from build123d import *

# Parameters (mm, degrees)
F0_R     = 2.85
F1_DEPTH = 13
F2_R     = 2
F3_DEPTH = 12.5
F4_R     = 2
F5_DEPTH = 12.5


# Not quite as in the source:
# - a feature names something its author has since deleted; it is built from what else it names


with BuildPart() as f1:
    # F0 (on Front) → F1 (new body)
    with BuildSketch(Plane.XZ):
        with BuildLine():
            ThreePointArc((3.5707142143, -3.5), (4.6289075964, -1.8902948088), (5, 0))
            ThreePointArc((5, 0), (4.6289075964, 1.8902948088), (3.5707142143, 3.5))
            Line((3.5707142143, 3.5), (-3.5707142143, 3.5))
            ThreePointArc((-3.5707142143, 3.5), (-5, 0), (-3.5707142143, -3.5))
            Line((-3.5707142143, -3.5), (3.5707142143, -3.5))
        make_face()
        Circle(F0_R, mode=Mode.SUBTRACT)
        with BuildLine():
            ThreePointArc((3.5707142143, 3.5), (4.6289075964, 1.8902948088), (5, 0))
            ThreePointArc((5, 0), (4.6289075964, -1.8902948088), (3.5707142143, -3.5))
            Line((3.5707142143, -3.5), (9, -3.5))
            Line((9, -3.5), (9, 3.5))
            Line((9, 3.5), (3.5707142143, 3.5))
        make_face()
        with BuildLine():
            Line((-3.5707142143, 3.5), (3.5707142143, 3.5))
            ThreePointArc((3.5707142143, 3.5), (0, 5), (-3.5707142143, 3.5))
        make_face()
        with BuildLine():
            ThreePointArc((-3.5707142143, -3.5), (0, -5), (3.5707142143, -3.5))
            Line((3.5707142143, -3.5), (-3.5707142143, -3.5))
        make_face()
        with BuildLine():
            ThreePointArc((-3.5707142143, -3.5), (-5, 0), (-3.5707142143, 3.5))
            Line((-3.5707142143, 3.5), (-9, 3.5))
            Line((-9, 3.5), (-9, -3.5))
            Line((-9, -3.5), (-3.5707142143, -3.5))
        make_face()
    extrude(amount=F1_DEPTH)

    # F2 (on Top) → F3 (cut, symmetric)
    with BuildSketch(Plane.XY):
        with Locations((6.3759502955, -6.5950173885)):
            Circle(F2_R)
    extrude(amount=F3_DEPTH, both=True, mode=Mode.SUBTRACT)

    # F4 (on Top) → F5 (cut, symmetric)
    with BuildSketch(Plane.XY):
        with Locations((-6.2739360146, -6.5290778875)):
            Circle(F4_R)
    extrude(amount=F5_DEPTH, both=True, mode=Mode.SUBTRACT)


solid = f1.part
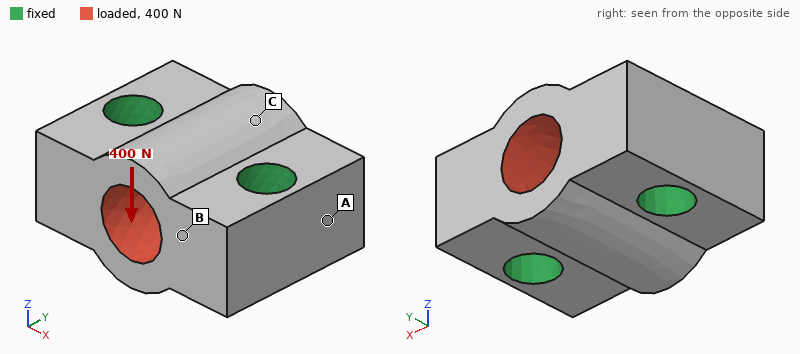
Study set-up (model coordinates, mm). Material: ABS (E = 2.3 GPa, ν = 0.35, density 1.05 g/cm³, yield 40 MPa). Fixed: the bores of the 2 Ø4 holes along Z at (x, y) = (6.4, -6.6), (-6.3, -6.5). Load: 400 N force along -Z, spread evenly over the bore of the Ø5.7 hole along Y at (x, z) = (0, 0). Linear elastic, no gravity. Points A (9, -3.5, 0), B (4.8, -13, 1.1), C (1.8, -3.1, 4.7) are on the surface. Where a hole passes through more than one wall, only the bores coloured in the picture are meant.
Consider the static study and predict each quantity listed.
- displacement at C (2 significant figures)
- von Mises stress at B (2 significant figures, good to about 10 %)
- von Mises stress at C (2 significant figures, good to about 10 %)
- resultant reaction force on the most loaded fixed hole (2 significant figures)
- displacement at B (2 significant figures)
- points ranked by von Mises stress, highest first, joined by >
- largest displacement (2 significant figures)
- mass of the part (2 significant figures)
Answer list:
15 µm
2.6 MPa
3.5 MPa
200 N
11 µm
C > B > A
23 µm
1.4 g
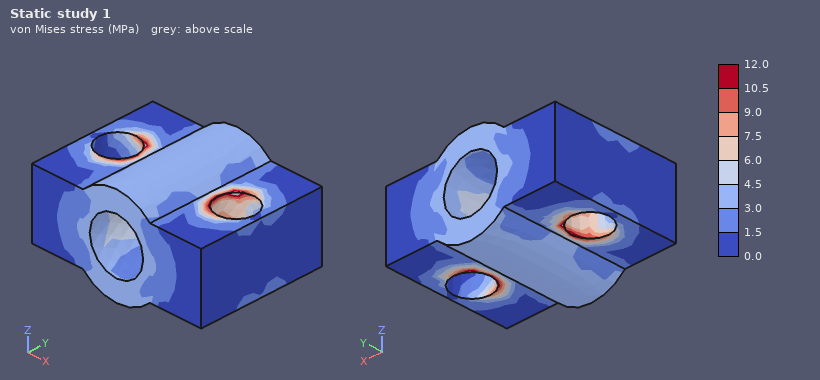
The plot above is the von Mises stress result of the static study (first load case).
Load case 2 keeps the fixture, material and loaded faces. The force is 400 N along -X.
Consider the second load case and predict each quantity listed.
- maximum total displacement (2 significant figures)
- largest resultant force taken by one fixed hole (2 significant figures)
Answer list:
10 µm
200 N
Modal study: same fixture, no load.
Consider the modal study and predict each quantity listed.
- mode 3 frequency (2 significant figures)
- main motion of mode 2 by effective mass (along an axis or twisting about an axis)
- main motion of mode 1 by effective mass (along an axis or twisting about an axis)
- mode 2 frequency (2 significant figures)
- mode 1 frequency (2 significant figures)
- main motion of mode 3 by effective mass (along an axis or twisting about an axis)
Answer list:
29 kHz
along Y
twisting about X
27 kHz
25 kHz
along Z
